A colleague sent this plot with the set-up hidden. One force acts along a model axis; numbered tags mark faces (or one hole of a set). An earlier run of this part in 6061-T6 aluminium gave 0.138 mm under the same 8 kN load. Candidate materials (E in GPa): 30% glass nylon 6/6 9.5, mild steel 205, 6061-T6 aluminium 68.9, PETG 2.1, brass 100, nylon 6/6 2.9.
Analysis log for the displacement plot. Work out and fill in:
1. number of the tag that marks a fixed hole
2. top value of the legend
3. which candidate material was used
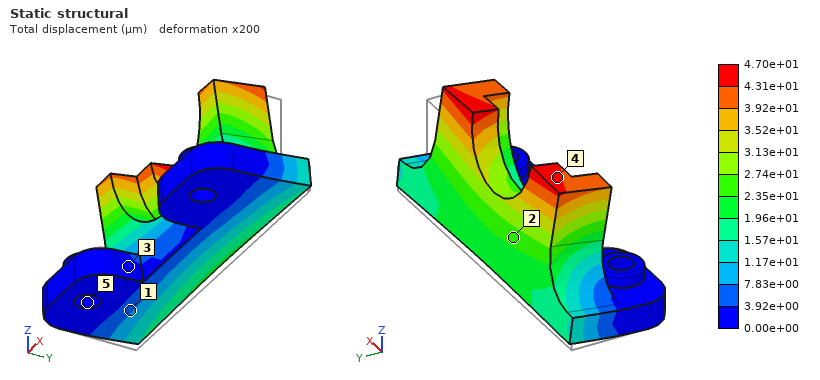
5
4.70e+01 µm
mild steel
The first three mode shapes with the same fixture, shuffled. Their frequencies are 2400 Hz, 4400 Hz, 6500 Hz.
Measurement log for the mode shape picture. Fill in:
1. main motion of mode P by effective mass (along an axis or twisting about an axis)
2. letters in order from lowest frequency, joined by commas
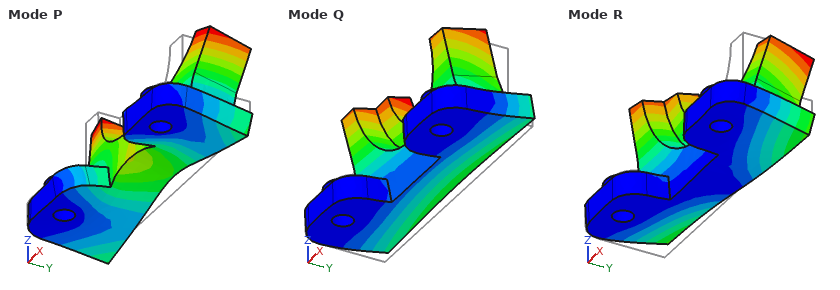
along Z
Q, R, P
